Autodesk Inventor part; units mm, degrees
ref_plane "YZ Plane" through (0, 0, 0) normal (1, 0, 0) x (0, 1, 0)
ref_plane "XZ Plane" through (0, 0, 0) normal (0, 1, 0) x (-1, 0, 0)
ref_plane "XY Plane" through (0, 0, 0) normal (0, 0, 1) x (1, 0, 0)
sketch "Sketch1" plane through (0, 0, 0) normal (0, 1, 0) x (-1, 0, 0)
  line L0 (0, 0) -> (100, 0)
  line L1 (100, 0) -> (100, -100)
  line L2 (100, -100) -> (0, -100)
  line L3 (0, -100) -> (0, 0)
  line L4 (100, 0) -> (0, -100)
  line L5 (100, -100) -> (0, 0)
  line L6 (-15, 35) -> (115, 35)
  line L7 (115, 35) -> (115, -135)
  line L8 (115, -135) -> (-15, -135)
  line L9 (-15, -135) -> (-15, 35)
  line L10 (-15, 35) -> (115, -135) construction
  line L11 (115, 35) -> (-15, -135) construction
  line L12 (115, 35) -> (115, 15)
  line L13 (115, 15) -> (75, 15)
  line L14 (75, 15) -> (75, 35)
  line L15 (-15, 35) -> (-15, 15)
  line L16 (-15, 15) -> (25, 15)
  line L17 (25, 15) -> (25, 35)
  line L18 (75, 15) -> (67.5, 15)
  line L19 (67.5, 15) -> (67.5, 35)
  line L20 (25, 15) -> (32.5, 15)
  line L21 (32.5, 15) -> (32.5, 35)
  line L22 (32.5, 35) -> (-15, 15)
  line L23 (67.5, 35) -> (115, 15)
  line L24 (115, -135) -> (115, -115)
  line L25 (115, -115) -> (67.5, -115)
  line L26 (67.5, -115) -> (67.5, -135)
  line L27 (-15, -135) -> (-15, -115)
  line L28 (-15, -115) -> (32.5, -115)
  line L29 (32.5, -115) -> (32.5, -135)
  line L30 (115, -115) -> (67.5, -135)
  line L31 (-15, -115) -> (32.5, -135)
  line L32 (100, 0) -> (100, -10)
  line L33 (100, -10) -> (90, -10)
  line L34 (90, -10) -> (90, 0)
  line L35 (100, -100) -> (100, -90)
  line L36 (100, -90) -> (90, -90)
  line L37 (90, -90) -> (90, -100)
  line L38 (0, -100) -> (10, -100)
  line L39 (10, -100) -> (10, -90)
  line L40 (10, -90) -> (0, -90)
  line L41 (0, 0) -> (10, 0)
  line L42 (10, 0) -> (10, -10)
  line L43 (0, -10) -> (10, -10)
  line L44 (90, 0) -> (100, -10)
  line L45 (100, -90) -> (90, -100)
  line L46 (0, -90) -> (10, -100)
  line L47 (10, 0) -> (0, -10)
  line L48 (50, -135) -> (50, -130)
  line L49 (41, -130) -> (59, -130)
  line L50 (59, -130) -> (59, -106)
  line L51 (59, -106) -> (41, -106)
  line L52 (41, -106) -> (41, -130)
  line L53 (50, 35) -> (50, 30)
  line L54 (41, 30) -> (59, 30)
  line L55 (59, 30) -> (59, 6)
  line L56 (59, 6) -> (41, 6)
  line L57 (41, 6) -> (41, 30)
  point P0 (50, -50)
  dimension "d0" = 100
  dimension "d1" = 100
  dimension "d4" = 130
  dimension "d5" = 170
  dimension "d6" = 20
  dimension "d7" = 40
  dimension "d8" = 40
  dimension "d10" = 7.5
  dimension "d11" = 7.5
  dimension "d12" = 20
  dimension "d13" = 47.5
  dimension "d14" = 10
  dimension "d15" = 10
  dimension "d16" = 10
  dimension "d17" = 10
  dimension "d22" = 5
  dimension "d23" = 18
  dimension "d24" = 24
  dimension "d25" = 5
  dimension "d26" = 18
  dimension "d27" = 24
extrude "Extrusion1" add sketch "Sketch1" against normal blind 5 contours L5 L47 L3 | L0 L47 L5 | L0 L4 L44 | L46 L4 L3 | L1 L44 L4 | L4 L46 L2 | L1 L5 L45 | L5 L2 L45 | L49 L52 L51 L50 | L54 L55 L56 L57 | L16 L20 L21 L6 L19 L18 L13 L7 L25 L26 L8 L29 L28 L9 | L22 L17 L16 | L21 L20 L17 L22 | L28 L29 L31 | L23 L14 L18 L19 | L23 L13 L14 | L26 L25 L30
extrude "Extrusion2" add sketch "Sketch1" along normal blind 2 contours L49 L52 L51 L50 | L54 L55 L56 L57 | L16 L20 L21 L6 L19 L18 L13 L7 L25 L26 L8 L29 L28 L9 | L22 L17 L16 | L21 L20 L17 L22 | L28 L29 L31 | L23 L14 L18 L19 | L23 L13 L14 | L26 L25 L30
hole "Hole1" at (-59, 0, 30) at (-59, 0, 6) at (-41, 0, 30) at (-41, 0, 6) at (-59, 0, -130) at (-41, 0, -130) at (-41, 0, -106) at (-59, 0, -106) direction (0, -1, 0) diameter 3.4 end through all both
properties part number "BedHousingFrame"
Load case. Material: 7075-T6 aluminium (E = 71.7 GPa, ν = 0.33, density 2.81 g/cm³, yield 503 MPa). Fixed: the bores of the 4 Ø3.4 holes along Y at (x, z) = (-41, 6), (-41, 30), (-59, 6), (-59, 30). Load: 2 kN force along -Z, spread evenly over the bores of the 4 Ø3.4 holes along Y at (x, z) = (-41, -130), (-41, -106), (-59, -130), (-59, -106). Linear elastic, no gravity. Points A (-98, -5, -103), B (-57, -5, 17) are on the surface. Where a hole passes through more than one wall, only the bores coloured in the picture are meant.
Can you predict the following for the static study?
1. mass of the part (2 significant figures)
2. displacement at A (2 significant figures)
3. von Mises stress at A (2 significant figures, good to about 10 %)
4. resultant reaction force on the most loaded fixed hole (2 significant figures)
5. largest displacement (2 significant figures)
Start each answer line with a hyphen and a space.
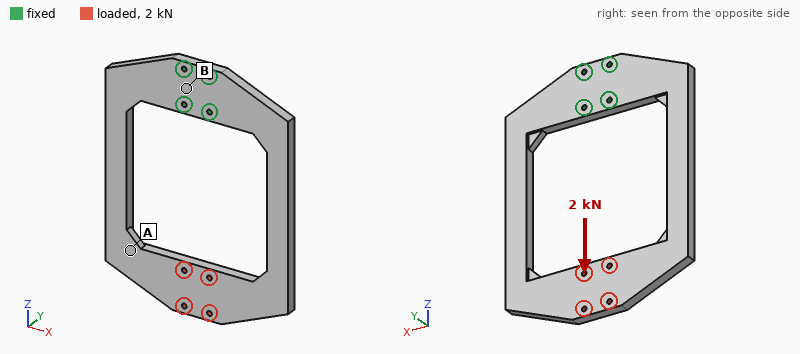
- 200 g
- 0.065 mm
- 14 MPa
- 1.6 kN
- 0.10 mm
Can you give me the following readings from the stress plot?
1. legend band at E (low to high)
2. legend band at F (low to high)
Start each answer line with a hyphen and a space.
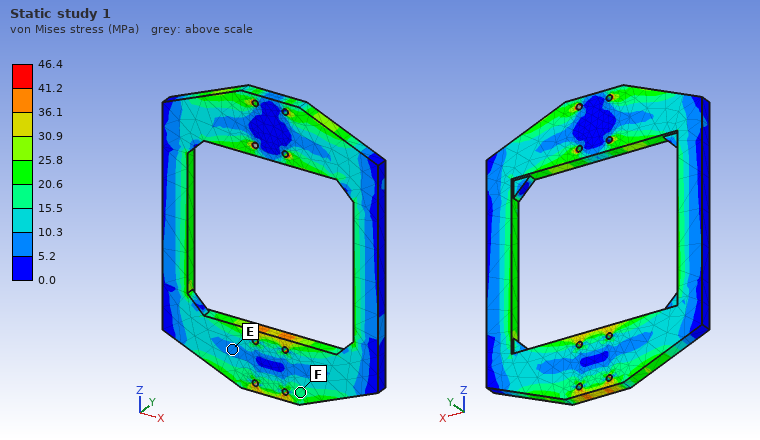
- 5.2 to 10.3 MPa
- 15.5 to 20.6 MPa
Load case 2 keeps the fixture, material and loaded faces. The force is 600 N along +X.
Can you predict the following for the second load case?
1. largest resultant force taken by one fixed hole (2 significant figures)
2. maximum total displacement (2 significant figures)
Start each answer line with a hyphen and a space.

- 1.6 kN
- 0.36 mm
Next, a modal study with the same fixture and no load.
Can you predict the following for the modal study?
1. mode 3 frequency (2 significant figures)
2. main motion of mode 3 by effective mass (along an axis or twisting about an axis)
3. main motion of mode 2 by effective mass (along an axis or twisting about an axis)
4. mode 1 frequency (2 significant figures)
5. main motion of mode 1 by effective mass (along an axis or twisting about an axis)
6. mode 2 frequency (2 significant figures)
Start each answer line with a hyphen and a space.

- 690 Hz
- along X
- twisting about Z
- 150 Hz
- along Y
- 410 Hz
